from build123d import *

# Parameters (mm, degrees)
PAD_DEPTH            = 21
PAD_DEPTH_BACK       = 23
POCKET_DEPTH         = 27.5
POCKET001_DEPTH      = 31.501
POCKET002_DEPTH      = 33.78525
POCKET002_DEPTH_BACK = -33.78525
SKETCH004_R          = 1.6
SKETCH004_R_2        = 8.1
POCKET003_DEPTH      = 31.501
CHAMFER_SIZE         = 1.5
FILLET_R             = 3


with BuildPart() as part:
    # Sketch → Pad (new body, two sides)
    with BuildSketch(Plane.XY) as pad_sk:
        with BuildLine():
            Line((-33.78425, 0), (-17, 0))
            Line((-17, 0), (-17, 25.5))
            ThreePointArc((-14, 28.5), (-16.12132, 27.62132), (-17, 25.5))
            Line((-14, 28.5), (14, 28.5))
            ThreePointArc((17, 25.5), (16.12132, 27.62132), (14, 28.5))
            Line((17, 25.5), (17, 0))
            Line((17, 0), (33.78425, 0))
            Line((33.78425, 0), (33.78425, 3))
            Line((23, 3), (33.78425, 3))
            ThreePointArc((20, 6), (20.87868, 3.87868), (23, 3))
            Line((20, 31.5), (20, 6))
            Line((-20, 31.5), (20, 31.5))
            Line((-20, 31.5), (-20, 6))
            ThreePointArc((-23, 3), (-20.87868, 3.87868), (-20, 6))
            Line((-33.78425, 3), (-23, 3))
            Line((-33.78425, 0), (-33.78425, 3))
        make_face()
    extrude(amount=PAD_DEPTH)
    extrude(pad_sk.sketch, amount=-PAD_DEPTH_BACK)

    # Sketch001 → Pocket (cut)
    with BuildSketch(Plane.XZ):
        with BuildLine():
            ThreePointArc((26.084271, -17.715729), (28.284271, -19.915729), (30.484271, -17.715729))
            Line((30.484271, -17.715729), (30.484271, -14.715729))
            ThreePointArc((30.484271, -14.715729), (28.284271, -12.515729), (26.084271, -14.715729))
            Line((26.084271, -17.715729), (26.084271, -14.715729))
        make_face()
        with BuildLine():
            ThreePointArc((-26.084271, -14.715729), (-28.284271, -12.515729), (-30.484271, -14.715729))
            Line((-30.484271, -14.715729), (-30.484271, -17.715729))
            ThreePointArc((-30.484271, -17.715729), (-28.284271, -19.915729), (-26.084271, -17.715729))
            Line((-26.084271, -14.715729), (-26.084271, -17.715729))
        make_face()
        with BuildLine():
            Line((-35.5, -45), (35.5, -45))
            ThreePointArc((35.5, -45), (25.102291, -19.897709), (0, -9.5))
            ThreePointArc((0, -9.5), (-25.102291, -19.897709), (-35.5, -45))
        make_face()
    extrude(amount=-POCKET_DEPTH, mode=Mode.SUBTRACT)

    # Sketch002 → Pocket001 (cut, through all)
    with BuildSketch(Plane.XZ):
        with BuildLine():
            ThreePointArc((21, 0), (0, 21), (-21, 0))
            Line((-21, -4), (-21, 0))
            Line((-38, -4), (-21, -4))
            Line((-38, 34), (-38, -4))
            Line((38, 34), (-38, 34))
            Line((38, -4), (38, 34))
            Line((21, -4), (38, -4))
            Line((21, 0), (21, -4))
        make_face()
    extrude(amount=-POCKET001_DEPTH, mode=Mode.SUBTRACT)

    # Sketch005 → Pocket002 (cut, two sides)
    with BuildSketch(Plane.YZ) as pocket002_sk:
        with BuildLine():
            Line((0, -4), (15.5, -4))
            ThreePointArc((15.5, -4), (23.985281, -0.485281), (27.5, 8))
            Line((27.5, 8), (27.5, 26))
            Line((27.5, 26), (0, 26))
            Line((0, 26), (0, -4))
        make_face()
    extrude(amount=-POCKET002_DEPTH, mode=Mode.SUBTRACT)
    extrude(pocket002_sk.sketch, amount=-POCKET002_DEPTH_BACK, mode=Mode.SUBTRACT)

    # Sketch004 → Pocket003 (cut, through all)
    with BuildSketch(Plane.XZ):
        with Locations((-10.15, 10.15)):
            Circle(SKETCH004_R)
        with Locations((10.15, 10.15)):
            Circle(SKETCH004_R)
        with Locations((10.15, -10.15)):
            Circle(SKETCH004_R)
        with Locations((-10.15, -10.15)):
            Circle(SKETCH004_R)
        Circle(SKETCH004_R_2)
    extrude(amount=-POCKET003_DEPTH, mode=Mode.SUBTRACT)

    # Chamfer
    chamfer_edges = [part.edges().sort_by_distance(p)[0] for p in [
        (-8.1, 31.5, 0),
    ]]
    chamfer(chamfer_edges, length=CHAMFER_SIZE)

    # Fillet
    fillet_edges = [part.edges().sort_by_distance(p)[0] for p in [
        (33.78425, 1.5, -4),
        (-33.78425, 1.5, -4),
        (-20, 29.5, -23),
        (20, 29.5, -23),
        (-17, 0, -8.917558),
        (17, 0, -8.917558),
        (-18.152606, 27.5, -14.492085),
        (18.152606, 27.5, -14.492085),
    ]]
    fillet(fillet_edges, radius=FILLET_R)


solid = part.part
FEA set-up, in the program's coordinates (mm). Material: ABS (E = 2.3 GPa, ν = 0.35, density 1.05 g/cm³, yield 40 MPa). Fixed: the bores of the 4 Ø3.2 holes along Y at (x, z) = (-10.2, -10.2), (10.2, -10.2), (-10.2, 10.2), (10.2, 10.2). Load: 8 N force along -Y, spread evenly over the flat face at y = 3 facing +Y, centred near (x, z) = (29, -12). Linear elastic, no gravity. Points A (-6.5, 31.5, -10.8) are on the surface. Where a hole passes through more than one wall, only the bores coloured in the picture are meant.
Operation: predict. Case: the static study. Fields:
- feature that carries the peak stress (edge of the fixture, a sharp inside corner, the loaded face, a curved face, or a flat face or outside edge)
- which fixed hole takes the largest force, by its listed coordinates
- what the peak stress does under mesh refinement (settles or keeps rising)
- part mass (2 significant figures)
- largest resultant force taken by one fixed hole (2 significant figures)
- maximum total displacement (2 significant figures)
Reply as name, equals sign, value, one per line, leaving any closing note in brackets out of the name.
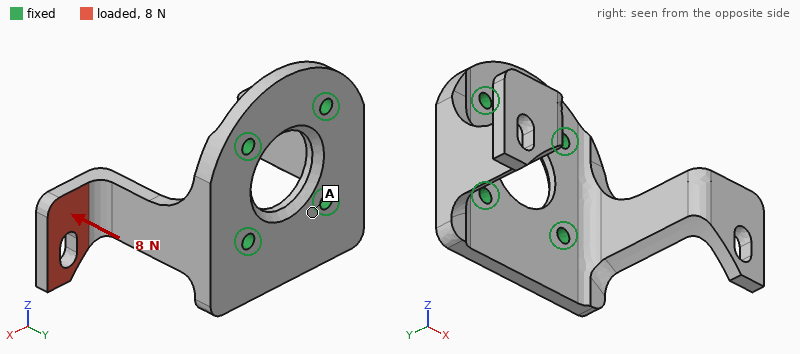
feature that carries the peak stress = edge of the fixture
which fixed hole takes the largest force, by its listed coordinates = (10.2, -10.2)
what the peak stress does under mesh refinement = keeps rising
part mass = 7.9 g
largest resultant force taken by one fixed hole = 9.3 N
maximum total displacement = 1.00 mm
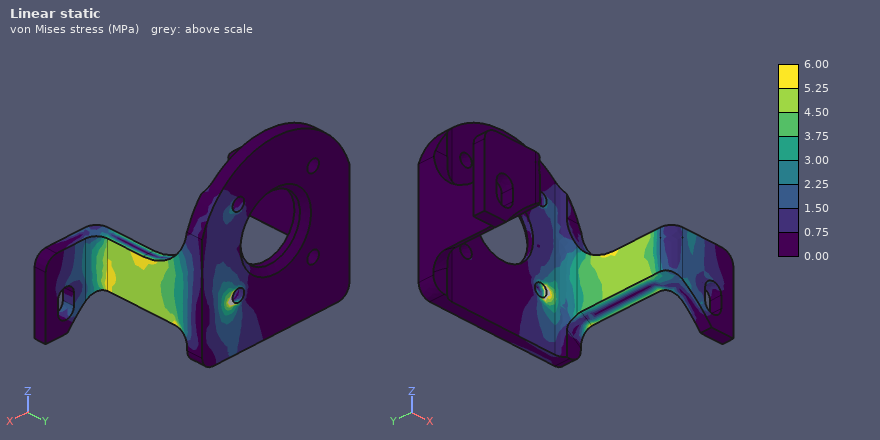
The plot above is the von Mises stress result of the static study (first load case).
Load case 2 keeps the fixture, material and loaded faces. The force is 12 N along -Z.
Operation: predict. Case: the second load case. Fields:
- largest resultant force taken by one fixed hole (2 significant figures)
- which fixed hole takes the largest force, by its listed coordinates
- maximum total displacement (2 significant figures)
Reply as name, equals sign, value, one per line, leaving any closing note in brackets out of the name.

largest resultant force taken by one fixed hole = 20 N
which fixed hole takes the largest force, by its listed coordinates = (10.2, 10.2)
maximum total displacement = 0.85 mm
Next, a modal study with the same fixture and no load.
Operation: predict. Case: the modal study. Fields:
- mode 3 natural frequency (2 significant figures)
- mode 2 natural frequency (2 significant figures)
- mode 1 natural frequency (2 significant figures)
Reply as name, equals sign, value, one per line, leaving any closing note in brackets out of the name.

mode 3 natural frequency = 910 Hz
mode 2 natural frequency = 410 Hz
mode 1 natural frequency = 410 Hz
